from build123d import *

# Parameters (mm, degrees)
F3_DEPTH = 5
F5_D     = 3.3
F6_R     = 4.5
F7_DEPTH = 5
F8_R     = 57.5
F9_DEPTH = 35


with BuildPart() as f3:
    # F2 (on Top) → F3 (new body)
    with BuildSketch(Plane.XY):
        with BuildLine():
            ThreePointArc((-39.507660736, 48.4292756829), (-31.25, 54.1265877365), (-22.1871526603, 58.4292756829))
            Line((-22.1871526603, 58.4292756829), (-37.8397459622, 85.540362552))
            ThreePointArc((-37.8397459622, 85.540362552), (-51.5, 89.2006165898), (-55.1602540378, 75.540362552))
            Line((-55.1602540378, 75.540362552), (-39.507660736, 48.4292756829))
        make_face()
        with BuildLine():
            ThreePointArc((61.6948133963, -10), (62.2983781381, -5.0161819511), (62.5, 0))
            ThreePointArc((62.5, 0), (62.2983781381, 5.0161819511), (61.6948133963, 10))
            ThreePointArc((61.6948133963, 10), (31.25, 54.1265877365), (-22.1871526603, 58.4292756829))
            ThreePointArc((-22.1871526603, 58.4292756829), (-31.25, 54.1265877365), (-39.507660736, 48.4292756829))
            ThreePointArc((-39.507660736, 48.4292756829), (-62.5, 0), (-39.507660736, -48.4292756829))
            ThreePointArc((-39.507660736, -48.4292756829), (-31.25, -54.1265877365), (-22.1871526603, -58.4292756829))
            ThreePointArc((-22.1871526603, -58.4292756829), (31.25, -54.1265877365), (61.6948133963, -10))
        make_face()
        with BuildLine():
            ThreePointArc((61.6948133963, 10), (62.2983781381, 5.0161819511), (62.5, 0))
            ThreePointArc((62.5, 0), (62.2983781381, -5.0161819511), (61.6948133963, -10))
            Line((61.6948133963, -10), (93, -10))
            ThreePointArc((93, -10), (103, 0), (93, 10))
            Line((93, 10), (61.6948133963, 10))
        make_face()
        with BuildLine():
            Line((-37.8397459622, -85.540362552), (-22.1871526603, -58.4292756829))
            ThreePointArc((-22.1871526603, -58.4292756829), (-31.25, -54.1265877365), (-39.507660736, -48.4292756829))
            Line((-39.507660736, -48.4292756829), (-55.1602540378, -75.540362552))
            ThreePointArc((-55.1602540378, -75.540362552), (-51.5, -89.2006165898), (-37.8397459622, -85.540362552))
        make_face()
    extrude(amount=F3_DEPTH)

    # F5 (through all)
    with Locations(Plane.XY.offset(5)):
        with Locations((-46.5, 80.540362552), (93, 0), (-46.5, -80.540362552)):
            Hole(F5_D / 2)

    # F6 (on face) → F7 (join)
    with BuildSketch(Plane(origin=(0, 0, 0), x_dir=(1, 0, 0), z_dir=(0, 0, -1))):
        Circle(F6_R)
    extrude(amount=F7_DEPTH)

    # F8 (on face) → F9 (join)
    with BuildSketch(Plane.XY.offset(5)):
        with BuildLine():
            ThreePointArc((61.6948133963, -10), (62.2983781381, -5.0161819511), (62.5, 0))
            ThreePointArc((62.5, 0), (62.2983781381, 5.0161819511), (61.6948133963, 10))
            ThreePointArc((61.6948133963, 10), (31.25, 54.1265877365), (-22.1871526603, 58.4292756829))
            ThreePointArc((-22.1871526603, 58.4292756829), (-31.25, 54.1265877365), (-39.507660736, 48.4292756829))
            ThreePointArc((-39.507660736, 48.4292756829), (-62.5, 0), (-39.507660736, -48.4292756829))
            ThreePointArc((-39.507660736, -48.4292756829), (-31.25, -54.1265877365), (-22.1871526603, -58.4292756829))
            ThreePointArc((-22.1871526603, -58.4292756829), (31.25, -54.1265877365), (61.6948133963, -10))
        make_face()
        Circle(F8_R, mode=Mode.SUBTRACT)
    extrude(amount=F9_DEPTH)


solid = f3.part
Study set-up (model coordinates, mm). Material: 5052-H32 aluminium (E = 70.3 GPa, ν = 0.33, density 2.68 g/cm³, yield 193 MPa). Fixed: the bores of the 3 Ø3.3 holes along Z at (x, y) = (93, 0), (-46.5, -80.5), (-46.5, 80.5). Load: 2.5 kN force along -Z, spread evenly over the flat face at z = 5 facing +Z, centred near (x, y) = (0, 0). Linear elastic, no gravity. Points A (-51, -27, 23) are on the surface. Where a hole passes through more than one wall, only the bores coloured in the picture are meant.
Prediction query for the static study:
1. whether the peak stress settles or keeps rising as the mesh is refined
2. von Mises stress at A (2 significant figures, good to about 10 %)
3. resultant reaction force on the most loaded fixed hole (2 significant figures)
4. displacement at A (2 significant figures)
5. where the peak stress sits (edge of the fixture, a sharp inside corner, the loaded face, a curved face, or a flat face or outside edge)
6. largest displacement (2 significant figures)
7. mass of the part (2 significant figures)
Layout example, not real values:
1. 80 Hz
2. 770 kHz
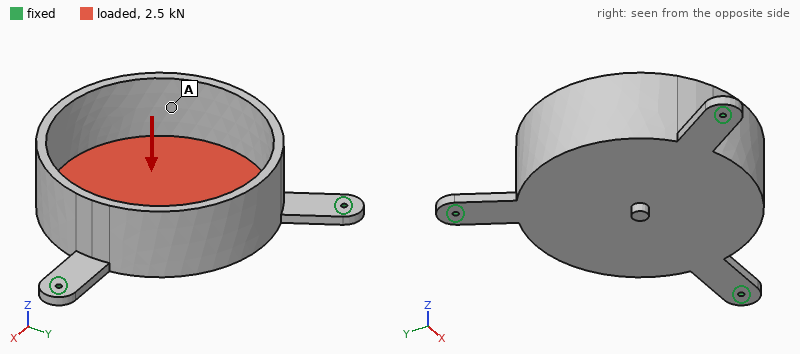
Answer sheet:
1. keeps rising
2. 14 MPa
3. 900 N
4. 0.25 mm
5. edge of the fixture
6. 0.34 mm
7. 370 g
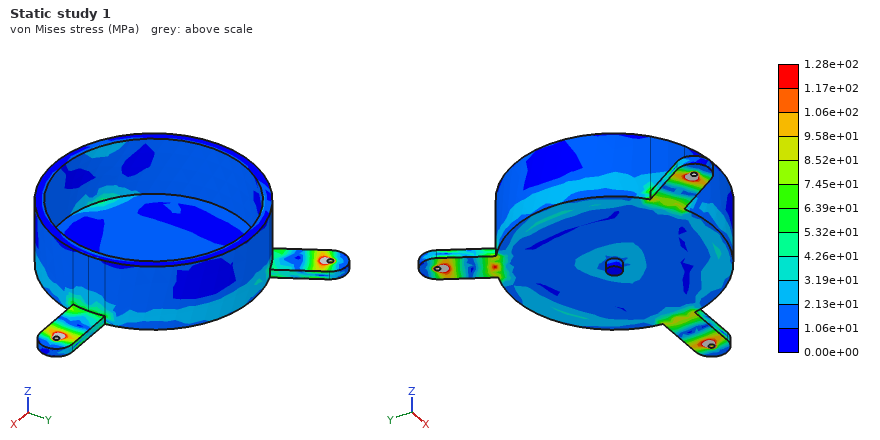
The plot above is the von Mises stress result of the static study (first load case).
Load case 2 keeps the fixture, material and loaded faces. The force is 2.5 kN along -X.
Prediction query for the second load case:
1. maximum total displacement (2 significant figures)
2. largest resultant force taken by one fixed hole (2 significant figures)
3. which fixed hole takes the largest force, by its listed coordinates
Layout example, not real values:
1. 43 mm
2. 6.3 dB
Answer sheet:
1. 36 µm
2. 1.5 kN
3. (93, 0)
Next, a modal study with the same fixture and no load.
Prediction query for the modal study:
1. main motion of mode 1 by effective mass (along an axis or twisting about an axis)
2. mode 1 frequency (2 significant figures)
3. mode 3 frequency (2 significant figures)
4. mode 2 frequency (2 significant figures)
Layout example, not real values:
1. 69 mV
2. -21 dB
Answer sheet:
1. along Z
2. 840 Hz
3. 990 Hz
4. 990 Hz
